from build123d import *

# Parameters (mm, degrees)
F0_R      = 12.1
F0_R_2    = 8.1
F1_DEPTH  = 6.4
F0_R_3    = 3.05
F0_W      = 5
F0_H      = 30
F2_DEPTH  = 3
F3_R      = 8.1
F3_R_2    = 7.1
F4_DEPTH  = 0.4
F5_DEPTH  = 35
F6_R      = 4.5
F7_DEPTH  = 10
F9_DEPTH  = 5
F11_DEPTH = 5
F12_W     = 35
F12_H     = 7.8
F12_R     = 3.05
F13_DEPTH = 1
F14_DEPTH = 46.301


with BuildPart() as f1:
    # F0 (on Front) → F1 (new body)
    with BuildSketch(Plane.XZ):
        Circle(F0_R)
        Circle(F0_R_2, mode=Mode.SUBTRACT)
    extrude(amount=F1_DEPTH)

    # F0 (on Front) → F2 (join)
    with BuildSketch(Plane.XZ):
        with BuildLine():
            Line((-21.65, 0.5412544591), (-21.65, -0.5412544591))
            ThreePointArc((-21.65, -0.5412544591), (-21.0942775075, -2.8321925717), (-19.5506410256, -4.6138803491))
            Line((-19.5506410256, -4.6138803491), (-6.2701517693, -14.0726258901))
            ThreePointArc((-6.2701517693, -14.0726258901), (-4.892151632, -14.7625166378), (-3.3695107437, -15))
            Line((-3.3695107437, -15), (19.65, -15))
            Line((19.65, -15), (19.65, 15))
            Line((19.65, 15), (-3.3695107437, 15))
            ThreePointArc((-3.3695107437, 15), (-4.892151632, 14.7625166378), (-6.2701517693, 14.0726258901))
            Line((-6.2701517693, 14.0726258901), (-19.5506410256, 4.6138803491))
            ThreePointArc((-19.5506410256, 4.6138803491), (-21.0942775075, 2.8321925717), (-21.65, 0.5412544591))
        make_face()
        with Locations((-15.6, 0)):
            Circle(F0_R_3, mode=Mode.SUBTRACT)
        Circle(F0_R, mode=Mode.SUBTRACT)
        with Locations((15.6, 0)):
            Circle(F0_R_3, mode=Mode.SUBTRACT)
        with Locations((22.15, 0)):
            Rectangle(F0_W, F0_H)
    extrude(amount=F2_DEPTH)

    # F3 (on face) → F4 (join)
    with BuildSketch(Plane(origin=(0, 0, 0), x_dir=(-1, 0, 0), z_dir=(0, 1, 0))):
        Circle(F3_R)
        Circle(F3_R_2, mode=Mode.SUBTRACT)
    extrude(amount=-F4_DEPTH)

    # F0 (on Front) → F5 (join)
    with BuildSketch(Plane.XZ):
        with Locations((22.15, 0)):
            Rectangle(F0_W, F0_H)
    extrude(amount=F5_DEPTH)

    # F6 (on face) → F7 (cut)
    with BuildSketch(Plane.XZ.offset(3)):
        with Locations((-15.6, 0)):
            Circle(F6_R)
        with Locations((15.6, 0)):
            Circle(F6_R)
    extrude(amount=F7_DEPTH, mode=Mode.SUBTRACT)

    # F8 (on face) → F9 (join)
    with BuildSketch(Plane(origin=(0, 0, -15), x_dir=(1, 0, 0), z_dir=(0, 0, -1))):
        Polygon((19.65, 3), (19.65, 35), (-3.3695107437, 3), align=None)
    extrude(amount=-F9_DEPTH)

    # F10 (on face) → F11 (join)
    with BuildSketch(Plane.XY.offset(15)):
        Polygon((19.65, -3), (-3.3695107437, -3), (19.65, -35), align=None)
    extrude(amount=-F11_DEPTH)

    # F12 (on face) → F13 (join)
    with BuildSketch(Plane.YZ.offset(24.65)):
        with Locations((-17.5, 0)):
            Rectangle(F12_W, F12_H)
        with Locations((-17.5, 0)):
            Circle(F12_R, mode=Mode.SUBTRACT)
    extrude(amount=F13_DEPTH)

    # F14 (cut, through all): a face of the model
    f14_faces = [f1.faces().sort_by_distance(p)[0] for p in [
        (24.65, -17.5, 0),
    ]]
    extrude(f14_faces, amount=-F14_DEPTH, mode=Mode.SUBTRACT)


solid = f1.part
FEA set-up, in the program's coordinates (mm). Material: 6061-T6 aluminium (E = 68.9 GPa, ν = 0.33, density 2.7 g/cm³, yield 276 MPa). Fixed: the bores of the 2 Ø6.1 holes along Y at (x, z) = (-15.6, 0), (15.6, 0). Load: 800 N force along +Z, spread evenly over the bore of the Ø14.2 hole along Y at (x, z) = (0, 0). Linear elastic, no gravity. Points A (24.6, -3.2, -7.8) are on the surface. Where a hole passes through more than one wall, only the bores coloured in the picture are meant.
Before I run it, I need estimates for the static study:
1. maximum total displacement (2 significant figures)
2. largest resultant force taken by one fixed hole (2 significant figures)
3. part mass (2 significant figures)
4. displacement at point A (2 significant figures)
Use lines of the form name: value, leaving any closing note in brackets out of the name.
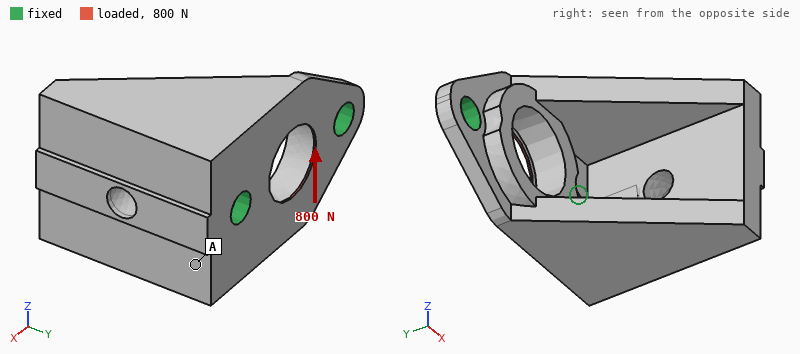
maximum total displacement: 7.9 µm
largest resultant force taken by one fixed hole: 410 N
part mass: 33 g
displacement at point A: 1.7 µm
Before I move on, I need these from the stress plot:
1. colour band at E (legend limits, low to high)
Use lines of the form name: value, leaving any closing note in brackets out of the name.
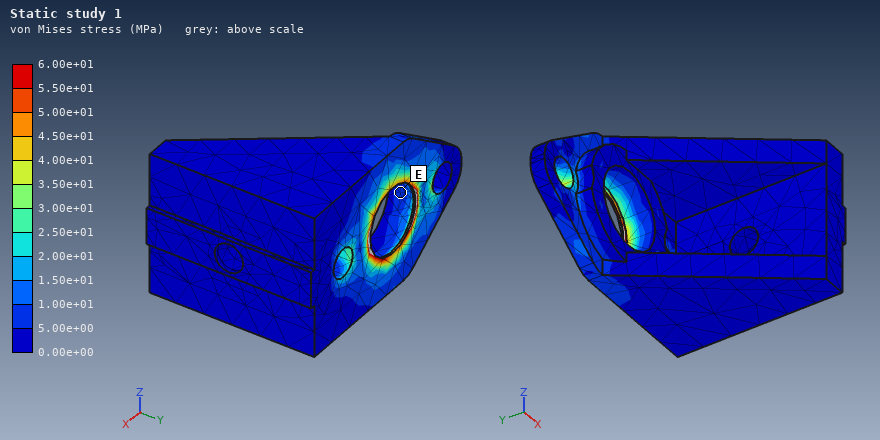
colour band at E: 5.00e+00 to 1.00e+01 MPa
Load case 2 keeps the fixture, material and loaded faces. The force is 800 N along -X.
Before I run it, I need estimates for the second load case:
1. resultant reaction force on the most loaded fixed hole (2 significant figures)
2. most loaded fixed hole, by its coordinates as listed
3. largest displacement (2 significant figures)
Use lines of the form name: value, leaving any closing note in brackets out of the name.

resultant reaction force on the most loaded fixed hole: 430 N
most loaded fixed hole, by its coordinates as listed: (15.6, 0)
largest displacement: 3.6 µm
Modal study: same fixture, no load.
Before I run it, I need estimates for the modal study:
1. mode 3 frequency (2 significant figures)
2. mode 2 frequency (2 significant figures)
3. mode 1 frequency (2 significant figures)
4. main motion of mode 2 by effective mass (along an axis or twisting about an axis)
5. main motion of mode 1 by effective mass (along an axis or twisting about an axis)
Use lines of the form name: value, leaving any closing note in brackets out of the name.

mode 3 frequency: 10 kHz
mode 2 frequency: 5500 Hz
mode 1 frequency: 3000 Hz
main motion of mode 2 by effective mass: along X
main motion of mode 1 by effective mass: along Z
